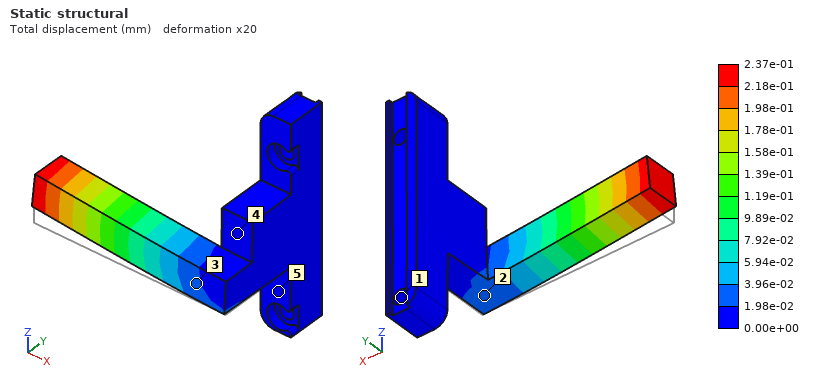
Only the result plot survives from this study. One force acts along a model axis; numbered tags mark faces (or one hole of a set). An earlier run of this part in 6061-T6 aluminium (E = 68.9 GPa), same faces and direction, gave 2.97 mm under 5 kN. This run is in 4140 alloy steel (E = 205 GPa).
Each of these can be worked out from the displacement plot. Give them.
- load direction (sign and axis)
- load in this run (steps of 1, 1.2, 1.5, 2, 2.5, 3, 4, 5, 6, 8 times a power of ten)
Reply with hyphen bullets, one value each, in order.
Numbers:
- +Z
- 1.2 kN
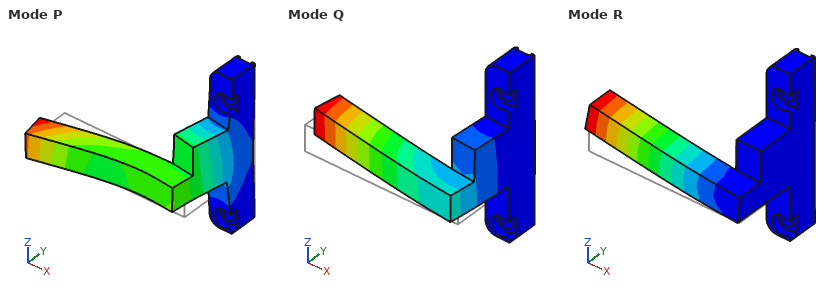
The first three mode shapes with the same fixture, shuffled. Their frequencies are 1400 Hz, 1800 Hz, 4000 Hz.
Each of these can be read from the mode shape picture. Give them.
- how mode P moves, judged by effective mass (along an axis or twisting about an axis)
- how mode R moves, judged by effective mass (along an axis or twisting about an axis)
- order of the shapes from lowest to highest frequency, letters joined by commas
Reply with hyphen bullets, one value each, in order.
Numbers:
- along X
- along Z
- Q, R, P
